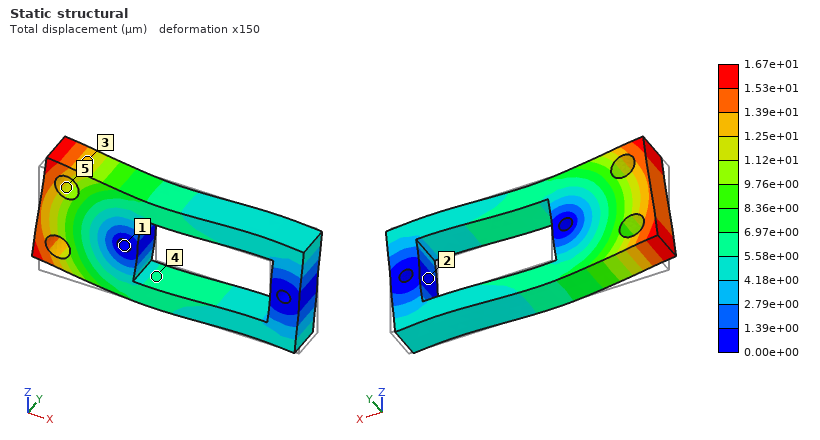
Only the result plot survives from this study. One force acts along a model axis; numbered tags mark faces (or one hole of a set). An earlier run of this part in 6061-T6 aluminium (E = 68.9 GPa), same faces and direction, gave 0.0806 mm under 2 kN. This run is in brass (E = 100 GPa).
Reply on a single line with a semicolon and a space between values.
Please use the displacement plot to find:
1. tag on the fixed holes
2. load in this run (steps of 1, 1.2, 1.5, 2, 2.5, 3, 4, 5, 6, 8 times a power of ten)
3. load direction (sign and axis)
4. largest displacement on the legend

1; 600 N; +Z; 1.67e+01 µm
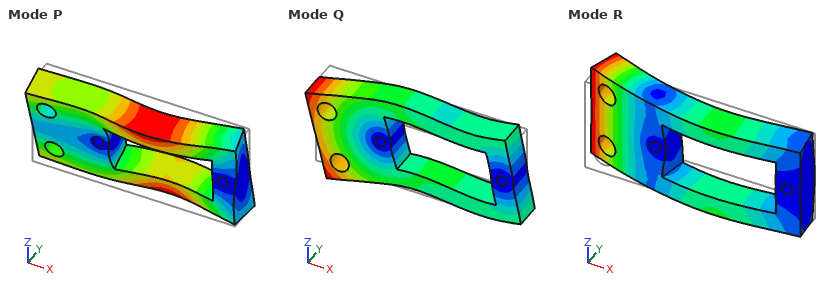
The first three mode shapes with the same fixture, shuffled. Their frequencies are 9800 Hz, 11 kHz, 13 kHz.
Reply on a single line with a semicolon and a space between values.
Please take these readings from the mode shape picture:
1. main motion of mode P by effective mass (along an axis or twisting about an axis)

twisting about X
